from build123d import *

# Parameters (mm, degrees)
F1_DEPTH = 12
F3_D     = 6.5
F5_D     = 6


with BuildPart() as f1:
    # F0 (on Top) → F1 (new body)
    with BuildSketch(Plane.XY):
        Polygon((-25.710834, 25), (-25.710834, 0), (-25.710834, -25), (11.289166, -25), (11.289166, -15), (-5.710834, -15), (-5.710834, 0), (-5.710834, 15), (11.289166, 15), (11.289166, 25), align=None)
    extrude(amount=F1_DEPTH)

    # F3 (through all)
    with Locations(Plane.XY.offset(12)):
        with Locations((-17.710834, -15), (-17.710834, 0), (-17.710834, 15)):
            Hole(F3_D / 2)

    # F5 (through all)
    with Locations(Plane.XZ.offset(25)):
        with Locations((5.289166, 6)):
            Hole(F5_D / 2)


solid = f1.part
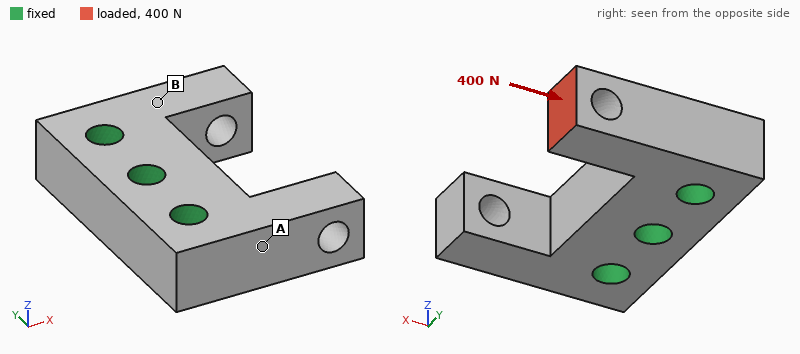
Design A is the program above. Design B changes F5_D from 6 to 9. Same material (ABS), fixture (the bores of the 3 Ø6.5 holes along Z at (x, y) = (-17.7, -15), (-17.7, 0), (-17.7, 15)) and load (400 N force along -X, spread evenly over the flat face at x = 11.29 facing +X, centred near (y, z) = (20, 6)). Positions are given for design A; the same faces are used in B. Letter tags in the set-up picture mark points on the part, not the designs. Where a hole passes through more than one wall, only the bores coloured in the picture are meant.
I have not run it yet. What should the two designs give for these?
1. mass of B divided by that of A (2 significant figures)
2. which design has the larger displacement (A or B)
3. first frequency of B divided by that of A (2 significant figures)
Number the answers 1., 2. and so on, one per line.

1. 0.95
2. B
3. 1.0
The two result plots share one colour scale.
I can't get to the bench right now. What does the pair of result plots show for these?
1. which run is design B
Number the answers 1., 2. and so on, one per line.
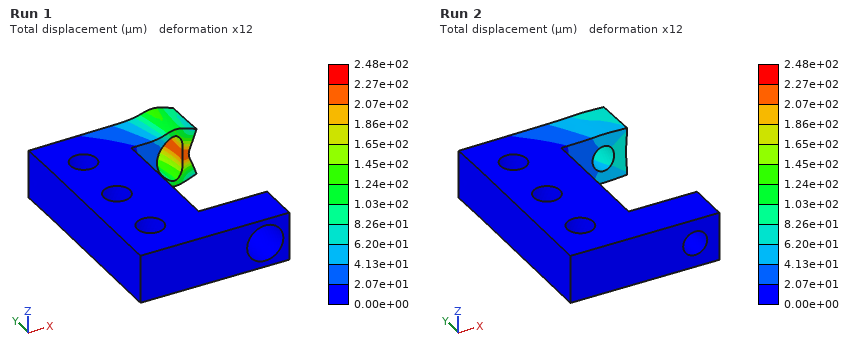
1. Run 1
